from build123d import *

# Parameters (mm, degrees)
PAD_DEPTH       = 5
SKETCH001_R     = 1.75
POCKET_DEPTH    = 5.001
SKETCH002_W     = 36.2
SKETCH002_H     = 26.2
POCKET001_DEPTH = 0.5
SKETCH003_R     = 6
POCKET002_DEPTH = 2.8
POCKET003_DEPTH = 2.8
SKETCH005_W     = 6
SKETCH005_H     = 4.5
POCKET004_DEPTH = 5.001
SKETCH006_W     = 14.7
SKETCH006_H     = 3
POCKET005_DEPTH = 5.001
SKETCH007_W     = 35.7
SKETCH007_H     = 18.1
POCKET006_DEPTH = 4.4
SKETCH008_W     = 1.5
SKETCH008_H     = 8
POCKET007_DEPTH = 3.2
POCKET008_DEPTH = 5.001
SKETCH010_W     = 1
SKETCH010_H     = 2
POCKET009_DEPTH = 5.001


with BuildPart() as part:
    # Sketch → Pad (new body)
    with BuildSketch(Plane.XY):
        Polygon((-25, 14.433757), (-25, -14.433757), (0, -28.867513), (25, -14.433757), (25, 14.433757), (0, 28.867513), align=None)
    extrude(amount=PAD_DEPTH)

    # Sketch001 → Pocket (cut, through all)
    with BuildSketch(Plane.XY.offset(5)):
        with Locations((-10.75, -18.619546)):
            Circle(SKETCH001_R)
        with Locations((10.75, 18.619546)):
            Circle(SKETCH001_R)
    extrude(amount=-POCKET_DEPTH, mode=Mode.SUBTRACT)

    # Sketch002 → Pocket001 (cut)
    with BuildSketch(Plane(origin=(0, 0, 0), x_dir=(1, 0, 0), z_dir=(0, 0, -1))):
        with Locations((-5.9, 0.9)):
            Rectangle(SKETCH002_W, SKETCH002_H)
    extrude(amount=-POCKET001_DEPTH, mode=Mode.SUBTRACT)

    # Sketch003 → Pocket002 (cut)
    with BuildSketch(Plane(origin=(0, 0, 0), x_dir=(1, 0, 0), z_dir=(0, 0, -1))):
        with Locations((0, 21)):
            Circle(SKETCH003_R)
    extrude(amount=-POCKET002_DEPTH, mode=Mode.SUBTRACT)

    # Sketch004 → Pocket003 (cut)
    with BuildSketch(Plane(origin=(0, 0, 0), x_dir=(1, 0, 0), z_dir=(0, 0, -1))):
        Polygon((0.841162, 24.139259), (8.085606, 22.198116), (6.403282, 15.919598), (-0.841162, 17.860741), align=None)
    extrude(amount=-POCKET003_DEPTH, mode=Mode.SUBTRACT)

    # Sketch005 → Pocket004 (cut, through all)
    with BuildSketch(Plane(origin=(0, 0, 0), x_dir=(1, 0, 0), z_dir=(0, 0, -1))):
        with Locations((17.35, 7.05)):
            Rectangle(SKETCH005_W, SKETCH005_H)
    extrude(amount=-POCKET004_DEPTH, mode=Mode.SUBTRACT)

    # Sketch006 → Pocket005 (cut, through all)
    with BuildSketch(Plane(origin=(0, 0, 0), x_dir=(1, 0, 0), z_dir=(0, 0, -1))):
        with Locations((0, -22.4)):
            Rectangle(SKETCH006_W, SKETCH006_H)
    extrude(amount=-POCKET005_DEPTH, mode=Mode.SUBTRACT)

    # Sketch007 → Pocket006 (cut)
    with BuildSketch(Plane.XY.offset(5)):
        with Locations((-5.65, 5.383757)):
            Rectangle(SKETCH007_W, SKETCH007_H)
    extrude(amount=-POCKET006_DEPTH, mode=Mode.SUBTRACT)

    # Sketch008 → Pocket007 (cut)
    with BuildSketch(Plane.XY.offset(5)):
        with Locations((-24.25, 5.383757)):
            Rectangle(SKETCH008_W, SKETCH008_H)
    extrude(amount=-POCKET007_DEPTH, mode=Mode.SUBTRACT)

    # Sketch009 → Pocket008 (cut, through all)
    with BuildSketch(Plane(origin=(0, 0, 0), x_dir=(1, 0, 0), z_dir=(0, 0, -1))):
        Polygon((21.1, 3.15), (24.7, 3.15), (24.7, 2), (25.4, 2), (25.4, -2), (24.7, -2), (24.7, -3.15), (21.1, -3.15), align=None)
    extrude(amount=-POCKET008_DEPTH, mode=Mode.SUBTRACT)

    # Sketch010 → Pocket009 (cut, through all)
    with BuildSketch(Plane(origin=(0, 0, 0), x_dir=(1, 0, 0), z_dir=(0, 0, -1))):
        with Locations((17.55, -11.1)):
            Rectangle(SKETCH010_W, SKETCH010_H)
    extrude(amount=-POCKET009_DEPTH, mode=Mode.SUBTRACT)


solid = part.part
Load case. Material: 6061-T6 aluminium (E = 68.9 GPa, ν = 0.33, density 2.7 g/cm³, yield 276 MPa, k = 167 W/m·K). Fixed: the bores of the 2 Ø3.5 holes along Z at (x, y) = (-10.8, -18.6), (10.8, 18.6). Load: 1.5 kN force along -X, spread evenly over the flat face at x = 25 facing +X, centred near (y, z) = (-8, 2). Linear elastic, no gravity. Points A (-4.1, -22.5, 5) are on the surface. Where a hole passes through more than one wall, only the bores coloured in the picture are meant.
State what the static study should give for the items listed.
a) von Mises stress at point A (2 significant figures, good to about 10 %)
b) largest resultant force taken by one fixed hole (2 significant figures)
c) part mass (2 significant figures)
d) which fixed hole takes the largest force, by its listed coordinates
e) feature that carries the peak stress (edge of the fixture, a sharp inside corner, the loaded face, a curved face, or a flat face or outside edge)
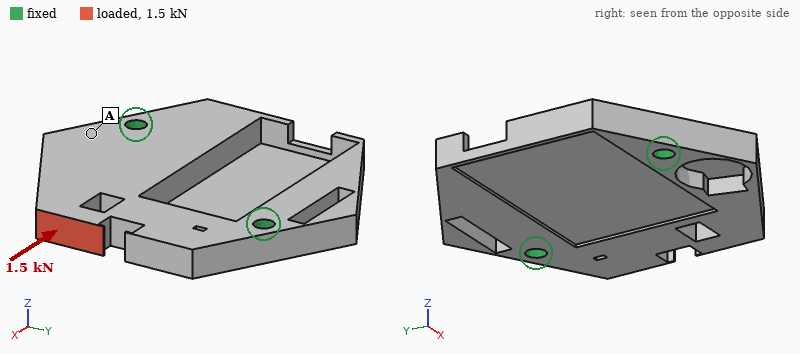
15 MPa
1.3 kN
18 g
(-10.8, -18.6)
the loaded face
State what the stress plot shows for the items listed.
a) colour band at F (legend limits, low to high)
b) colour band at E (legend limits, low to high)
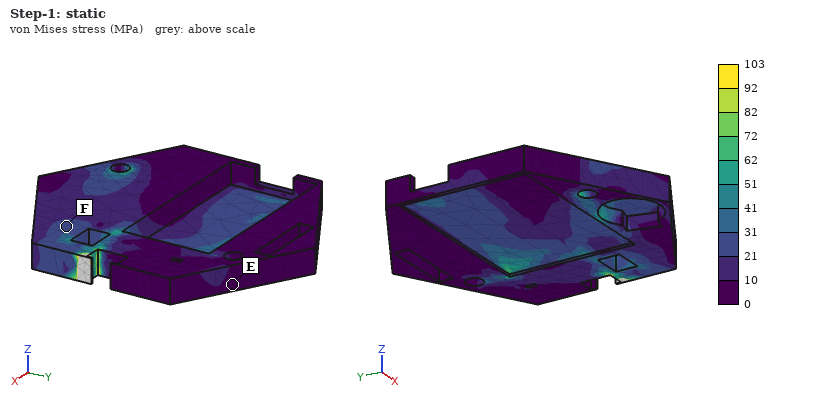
21 to 31 MPa
0 to 10 MPa
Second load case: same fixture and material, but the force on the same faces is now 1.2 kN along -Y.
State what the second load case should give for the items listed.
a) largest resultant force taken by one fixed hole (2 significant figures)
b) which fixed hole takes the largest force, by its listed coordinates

1.2 kN
(10.8, 18.6)
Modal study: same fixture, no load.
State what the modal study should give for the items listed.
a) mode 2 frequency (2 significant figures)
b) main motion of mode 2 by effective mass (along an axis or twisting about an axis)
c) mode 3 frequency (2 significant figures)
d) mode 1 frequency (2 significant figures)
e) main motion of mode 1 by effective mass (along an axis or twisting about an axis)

5200 Hz
along Z
11 kHz
4300 Hz
along Z
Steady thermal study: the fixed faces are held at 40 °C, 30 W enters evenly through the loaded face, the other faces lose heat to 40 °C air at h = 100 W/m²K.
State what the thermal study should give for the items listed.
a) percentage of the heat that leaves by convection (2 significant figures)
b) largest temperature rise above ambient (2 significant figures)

21 %
72 K
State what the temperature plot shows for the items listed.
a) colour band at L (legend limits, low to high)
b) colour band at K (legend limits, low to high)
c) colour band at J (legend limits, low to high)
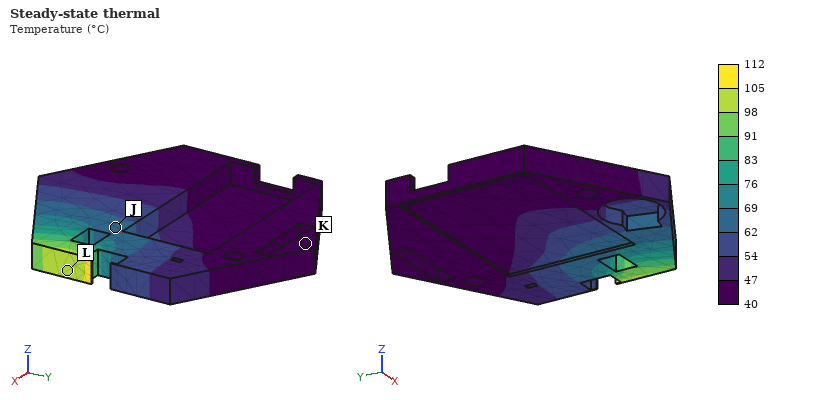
98 to 105 °C
40 to 47 °C
62 to 69 °C
